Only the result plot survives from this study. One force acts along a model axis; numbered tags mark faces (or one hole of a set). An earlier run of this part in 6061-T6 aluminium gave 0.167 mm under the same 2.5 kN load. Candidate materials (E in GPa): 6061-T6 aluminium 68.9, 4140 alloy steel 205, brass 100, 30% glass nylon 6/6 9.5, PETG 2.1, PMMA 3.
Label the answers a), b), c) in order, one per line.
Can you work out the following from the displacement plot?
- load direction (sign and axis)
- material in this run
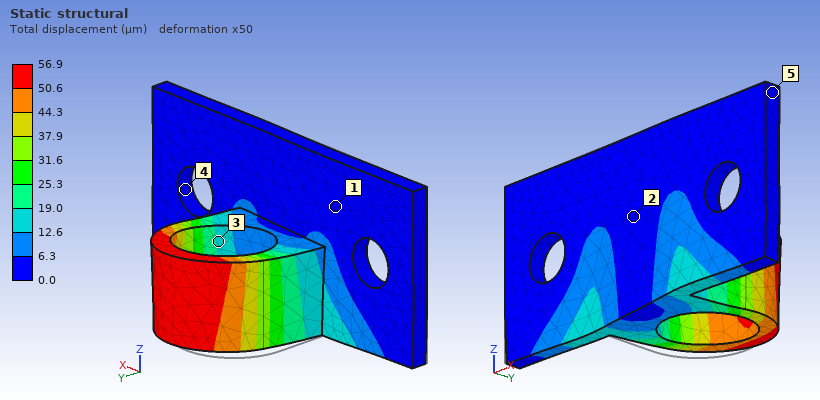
a) +X
b) 4140 alloy steel
